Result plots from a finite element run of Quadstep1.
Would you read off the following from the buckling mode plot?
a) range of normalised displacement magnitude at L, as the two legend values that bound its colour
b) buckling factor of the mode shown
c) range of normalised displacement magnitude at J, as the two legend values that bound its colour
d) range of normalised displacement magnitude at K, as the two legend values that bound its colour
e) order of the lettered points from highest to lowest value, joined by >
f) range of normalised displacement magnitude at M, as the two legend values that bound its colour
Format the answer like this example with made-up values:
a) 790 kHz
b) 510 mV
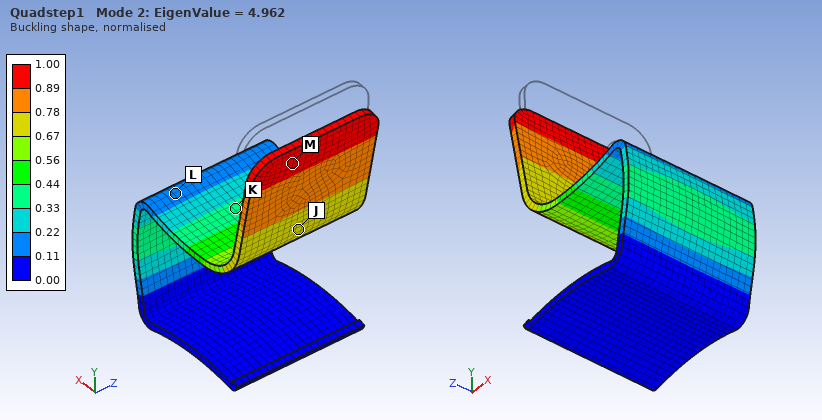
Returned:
a) 0.11 to 0.22
b) 4.962
c) 0.67 to 0.78
d) 0.33 to 0.44
e) M > J > K > L
f) 0.89 to 1.00
